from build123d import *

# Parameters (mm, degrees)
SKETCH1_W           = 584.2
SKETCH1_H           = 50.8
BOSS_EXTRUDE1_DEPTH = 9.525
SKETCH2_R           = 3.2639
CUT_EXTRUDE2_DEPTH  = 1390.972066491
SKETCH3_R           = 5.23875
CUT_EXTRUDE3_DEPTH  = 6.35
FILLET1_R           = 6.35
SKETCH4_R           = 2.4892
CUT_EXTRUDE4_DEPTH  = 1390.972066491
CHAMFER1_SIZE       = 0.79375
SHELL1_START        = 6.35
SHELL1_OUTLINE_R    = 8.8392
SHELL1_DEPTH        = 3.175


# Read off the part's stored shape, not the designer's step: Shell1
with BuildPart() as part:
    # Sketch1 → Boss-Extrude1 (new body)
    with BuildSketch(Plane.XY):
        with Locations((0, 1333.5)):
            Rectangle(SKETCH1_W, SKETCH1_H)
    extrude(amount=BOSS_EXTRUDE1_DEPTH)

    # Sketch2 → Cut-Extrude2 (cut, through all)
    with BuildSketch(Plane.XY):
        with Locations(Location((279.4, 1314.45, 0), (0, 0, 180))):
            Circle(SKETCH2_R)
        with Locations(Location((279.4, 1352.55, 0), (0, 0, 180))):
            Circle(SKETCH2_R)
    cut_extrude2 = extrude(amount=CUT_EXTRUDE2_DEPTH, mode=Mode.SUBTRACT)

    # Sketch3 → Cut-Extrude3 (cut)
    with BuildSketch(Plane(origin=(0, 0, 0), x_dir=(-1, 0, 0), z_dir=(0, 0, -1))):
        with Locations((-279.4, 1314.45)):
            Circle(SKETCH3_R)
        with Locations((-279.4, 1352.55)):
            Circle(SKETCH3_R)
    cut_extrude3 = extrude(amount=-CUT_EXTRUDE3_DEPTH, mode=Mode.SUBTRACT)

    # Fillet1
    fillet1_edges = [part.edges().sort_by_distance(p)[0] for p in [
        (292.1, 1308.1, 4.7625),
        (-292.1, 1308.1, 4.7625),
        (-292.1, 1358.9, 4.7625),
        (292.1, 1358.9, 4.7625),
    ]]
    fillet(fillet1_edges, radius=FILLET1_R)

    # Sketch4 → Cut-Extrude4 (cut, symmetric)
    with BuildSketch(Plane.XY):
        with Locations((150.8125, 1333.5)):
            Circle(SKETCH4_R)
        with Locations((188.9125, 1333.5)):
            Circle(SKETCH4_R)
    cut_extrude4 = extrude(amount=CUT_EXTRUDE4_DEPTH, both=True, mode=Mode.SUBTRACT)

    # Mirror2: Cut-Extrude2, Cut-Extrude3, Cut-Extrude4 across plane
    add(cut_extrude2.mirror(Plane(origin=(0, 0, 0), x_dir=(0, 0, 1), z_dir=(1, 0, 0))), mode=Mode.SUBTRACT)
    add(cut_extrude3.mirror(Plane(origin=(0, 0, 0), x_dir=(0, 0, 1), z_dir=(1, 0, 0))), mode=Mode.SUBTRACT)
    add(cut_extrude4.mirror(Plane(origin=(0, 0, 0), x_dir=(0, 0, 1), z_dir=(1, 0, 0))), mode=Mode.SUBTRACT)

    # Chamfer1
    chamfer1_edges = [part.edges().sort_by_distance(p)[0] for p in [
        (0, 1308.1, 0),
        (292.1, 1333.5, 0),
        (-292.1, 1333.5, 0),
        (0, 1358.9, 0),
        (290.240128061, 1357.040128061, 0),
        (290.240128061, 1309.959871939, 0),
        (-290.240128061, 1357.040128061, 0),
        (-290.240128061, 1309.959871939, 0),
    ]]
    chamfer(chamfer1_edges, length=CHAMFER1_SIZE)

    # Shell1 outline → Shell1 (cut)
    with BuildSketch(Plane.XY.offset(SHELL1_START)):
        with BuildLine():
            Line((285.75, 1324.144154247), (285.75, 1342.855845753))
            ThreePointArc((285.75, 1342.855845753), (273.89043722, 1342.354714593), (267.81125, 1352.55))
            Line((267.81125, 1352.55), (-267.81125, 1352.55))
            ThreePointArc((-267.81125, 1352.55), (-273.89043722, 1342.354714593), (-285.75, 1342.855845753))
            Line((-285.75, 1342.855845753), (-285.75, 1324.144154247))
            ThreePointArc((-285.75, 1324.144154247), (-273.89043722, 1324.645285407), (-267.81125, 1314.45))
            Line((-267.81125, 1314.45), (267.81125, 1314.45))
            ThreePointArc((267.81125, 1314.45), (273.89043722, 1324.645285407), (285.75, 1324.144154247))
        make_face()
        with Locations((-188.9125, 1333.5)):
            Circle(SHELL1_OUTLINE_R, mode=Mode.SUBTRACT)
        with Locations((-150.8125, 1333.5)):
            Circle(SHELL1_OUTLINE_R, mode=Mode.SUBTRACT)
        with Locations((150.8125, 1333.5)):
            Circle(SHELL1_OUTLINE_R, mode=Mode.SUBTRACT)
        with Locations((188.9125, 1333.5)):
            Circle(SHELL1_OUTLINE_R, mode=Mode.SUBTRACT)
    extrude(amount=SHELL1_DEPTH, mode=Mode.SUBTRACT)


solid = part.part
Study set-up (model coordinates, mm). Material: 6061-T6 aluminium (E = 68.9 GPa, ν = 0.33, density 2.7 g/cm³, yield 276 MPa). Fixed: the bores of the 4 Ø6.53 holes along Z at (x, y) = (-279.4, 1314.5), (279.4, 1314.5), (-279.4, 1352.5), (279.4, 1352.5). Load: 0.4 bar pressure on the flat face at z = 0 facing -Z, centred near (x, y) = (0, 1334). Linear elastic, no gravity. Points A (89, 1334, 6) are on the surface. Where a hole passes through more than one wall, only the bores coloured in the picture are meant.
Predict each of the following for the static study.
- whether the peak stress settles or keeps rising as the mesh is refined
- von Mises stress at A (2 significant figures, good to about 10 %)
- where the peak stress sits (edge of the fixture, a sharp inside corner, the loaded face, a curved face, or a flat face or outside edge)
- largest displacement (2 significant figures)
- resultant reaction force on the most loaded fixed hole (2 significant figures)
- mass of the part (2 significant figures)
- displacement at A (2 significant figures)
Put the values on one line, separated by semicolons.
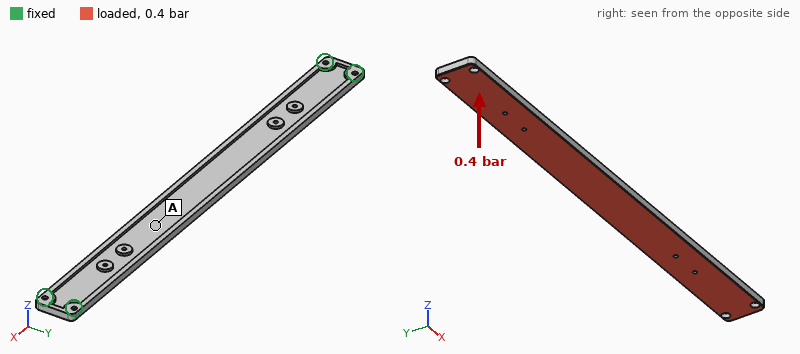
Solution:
keeps rising; 21 MPa; edge of the fixture; 4.3 mm; 1.2 kN; 580 g; 3.5 mm
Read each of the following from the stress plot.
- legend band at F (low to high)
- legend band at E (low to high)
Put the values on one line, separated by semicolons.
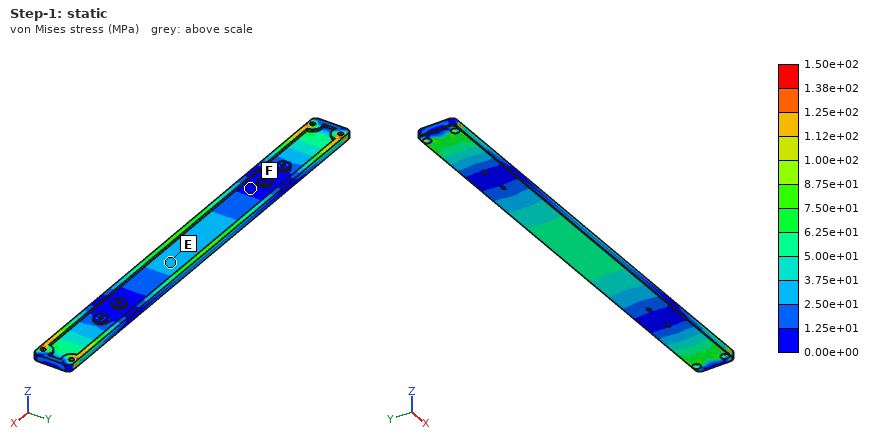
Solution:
0.00e+00 to 1.25e+01 MPa; 2.50e+01 to 3.75e+01 MPa
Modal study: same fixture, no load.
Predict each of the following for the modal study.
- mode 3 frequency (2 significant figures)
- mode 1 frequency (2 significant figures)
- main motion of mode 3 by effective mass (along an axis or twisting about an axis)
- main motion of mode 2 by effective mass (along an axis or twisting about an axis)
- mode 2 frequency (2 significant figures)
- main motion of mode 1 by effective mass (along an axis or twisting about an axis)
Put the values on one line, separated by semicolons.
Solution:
660 Hz; 120 Hz; along Y; twisting about Y; 340 Hz; along Z
